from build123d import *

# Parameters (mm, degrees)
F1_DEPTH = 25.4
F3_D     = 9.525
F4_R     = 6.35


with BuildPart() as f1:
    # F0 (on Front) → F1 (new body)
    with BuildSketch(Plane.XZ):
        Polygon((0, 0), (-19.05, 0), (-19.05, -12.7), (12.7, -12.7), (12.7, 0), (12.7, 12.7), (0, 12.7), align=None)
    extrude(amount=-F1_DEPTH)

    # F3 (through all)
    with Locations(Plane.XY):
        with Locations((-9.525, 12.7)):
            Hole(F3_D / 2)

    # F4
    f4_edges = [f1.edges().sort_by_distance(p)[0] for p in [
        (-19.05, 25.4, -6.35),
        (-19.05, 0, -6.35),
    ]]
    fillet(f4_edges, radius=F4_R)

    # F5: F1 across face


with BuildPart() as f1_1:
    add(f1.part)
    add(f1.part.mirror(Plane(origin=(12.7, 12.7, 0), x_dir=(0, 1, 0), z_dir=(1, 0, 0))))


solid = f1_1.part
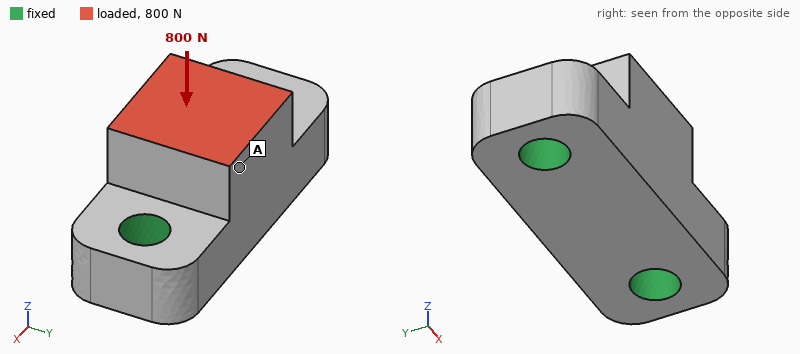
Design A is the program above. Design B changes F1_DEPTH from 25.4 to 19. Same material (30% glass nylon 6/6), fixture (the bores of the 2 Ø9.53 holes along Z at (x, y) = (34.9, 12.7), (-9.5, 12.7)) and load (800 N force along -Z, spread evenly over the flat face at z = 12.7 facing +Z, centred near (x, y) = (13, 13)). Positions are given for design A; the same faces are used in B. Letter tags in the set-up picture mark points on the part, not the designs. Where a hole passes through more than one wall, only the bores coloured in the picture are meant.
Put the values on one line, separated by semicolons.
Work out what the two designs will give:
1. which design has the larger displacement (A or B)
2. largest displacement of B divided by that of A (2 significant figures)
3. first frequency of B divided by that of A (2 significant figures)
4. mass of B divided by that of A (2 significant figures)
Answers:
B; 1.6; 0.97; 0.73
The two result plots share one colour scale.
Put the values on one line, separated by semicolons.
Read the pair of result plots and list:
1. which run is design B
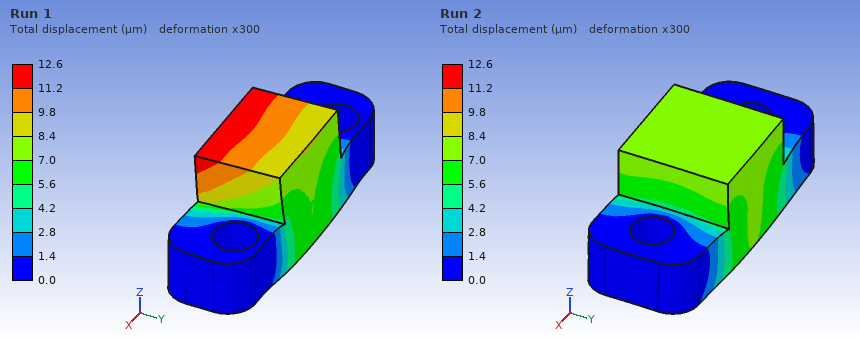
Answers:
Run 1
